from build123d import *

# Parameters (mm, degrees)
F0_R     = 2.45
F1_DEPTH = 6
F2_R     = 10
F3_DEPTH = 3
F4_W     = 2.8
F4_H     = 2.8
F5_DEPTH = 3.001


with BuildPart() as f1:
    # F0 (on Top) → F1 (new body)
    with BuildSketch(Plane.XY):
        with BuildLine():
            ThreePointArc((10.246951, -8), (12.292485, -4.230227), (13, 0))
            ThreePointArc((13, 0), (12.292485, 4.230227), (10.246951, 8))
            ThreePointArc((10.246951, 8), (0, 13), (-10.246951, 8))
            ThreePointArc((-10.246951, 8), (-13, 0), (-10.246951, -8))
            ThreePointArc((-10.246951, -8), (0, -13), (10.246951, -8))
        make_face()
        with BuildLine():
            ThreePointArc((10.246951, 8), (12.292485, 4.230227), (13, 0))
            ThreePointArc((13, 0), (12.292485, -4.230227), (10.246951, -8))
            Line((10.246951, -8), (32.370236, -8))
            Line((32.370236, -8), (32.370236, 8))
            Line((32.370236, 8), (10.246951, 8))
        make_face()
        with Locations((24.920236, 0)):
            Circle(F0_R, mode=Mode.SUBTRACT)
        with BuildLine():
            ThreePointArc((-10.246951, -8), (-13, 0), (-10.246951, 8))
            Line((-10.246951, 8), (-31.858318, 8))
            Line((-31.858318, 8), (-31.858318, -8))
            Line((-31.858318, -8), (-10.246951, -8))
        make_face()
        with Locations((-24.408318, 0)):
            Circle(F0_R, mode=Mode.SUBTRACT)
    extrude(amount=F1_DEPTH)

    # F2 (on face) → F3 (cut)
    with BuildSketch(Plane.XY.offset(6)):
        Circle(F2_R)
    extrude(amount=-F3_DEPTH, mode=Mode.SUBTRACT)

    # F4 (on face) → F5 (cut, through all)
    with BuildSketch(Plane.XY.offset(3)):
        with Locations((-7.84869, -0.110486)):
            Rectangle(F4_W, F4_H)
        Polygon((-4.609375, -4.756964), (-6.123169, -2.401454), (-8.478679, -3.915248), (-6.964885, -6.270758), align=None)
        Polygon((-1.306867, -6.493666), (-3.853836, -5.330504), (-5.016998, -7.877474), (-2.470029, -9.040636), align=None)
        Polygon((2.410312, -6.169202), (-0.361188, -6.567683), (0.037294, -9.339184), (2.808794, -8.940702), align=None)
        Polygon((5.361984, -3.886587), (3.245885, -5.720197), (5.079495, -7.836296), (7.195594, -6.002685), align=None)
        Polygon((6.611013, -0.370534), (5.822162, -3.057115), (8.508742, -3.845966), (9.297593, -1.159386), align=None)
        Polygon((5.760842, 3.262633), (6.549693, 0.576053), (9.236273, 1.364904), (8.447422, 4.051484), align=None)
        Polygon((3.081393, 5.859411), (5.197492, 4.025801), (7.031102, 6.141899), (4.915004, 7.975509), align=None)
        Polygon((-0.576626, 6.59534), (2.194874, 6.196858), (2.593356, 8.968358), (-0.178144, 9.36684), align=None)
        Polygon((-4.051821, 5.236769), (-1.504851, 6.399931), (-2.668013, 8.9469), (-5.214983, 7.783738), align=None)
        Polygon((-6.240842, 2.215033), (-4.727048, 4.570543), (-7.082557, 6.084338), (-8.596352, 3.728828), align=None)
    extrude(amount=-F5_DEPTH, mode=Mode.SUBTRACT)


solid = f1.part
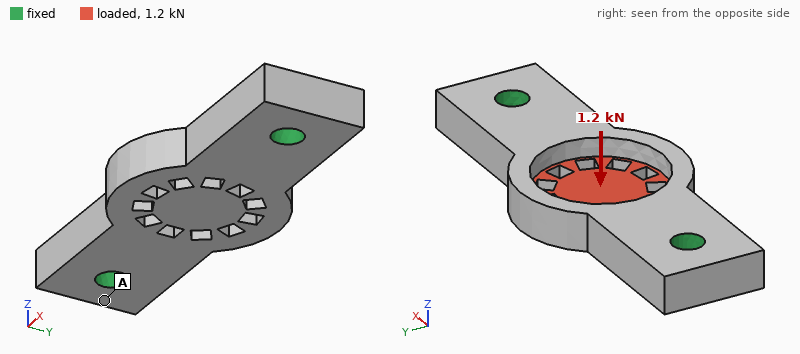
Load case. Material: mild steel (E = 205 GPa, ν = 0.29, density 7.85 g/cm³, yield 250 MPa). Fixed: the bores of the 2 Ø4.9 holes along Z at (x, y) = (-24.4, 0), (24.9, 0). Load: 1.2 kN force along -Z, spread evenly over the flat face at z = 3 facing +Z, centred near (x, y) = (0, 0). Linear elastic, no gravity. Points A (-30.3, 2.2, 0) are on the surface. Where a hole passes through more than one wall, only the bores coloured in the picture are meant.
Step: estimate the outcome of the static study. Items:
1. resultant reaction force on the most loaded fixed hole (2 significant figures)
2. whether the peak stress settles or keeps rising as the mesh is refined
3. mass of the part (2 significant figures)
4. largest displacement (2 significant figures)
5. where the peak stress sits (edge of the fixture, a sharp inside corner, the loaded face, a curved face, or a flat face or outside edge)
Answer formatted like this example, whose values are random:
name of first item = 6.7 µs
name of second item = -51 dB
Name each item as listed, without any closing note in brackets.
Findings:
resultant reaction force on the most loaded fixed hole = 730 N
whether the peak stress settles or keeps rising as the mesh is refined = keeps rising
mass of the part = 44 g
largest displacement = 18 µm
where the peak stress sits = edge of the fixture
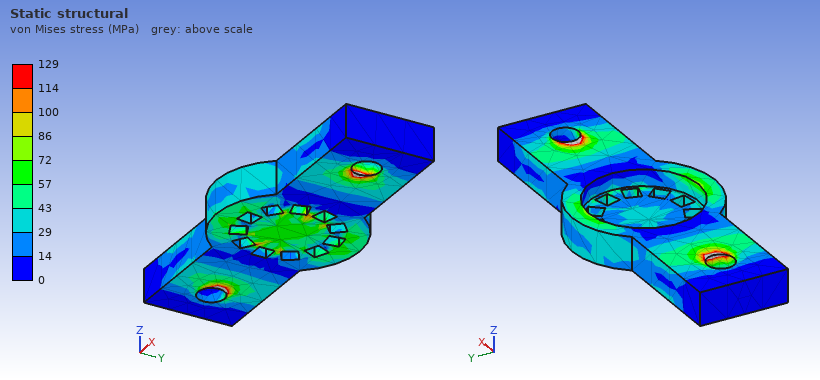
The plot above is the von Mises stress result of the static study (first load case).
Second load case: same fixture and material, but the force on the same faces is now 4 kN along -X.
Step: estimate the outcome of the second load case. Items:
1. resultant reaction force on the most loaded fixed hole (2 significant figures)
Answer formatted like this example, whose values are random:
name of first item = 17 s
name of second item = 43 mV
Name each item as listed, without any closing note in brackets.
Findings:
resultant reaction force on the most loaded fixed hole = 2.0 kN
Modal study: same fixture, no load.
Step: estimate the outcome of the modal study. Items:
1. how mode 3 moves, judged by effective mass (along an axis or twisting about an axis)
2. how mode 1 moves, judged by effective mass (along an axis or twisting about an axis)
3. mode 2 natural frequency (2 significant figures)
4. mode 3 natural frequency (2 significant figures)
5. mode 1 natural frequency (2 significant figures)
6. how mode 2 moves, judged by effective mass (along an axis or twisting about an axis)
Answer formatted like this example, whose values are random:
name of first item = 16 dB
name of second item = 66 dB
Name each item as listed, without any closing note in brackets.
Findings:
how mode 3 moves, judged by effective mass = along Y
how mode 1 moves, judged by effective mass = along Z
mode 2 natural frequency = 14 kHz
mode 3 natural frequency = 22 kHz
mode 1 natural frequency = 12 kHz
how mode 2 moves, judged by effective mass = twisting about X
